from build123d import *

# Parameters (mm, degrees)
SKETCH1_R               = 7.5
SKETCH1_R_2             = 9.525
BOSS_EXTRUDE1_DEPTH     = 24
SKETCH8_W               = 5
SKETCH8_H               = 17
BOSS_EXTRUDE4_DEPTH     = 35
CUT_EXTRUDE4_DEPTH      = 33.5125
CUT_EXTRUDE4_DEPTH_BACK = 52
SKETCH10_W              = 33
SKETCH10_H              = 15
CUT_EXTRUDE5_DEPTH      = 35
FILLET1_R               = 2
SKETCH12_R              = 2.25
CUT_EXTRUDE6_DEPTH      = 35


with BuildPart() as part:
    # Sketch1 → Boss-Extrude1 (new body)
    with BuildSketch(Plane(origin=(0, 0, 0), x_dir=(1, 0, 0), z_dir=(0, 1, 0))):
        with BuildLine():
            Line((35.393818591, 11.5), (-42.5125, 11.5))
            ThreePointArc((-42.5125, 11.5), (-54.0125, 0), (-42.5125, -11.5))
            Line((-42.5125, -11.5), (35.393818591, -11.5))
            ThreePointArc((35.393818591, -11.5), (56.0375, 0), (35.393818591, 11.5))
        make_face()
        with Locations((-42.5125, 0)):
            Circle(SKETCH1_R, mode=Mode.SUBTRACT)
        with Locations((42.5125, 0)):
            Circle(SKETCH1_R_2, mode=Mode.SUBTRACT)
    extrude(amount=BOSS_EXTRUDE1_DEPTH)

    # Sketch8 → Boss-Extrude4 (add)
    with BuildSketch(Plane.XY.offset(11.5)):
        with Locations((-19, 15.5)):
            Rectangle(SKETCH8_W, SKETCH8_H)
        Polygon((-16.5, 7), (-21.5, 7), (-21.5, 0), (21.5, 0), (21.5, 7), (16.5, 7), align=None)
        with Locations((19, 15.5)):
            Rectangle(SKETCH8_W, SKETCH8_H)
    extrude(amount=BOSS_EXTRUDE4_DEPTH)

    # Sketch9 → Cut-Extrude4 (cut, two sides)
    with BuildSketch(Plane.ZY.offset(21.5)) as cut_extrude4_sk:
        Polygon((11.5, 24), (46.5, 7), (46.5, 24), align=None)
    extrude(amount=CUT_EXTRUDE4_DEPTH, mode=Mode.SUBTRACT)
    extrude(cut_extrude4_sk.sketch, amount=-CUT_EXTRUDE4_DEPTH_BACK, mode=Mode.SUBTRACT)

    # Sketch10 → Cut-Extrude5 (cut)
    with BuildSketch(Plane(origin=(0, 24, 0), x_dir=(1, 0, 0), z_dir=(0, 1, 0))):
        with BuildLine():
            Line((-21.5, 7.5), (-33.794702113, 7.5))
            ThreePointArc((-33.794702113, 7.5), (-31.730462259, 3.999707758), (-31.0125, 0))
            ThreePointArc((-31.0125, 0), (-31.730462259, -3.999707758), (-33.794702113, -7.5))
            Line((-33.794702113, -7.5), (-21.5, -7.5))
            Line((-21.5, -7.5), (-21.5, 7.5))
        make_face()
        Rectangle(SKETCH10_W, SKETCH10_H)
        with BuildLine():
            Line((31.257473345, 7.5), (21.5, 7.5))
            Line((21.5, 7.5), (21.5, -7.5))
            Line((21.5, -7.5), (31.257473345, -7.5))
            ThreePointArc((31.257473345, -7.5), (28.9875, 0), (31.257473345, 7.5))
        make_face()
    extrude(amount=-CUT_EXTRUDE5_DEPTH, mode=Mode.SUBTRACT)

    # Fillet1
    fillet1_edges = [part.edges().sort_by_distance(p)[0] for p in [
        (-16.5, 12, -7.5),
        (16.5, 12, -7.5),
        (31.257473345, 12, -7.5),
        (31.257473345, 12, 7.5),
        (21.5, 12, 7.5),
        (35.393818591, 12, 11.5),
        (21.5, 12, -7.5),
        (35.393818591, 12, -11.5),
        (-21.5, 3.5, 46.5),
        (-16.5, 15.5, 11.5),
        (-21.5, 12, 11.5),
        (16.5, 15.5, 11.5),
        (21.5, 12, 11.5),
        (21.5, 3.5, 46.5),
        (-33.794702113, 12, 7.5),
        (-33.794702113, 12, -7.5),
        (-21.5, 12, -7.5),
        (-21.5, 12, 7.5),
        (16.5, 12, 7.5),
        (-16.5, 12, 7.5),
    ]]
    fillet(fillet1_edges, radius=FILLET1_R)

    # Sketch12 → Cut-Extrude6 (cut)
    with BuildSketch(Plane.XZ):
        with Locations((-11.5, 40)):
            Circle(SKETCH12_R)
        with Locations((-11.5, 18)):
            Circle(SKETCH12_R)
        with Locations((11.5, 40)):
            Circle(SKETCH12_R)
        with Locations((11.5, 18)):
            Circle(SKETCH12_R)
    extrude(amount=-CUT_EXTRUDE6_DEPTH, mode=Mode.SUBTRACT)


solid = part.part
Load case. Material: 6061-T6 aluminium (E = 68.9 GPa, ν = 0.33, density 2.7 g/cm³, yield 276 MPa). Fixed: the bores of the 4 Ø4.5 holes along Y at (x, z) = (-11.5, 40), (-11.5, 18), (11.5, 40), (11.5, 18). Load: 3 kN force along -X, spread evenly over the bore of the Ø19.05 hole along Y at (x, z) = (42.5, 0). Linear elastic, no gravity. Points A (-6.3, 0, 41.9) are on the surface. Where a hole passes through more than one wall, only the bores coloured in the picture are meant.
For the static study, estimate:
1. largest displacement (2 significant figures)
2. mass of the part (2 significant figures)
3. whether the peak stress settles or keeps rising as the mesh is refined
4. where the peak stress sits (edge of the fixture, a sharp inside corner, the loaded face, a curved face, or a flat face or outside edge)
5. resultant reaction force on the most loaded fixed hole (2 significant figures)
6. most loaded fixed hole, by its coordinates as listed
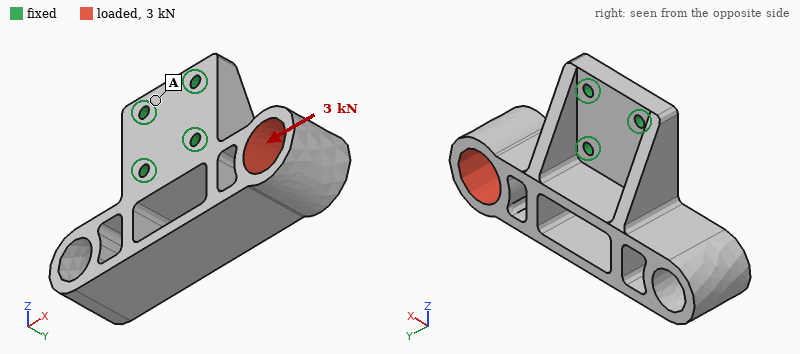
0.12 mm
120 g
keeps rising
edge of the fixture
2.3 kN
(11.5, 18)
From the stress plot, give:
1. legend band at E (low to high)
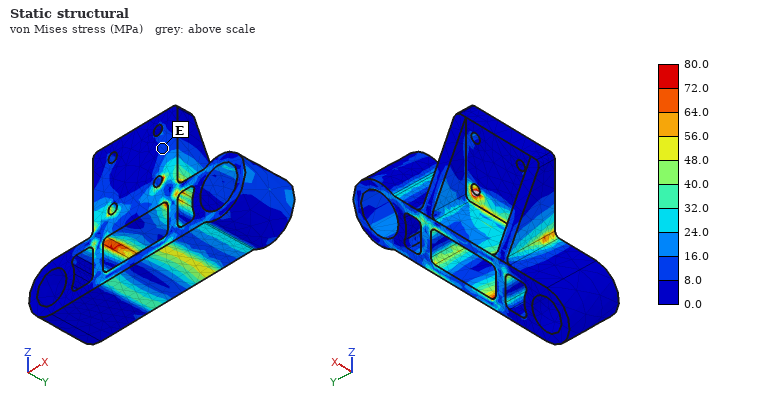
8.0 to 16.0 MPa
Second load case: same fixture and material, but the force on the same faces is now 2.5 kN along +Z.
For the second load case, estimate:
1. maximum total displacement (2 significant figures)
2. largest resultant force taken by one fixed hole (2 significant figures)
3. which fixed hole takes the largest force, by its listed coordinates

0.31 mm
2.4 kN
(11.5, 18)
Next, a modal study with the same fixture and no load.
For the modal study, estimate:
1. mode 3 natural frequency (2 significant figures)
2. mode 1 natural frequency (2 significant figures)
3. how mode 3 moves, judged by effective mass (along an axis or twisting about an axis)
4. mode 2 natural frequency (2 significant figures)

3900 Hz
2700 Hz
along Y
2900 Hz
